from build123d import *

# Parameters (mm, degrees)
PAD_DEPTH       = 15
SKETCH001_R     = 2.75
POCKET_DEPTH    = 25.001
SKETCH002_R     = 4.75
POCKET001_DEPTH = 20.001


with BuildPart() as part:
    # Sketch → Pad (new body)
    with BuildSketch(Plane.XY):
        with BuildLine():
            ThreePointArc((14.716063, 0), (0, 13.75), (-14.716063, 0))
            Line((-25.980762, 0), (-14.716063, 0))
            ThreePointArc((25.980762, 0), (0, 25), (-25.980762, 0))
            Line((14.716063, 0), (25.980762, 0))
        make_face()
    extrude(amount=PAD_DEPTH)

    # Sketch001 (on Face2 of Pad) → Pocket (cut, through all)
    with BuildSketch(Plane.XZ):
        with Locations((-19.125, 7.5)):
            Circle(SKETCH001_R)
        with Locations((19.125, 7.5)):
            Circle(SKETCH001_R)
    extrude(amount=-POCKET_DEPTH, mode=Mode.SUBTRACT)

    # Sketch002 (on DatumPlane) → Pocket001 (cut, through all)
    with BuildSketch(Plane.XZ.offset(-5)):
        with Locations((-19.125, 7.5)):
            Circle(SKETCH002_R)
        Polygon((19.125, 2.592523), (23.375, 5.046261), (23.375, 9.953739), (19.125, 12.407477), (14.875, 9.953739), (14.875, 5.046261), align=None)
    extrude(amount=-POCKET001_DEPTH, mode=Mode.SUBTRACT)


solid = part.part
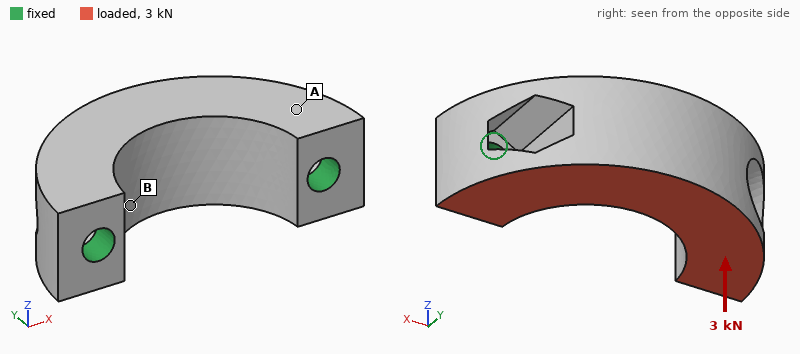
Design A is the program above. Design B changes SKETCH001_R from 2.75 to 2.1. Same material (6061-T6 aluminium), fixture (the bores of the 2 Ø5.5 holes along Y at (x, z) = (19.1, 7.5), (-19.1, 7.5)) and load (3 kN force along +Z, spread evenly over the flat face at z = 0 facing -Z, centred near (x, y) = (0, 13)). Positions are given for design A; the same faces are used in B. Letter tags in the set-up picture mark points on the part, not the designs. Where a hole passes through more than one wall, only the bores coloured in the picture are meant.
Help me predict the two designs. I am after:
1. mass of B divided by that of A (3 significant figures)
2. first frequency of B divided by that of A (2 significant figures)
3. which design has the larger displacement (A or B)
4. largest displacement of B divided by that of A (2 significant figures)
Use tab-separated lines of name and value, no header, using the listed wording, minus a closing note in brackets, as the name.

mass of B divided by that of A	1.01
first frequency of B divided by that of A	0.86
which design has the larger displacement	B
largest displacement of B divided by that of A	1.3
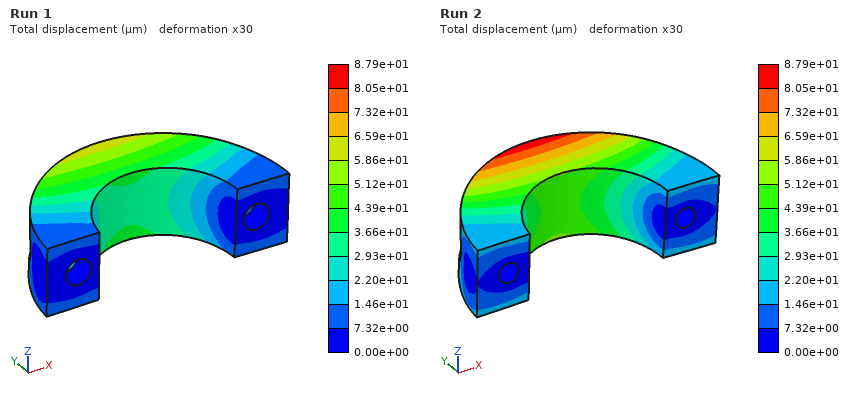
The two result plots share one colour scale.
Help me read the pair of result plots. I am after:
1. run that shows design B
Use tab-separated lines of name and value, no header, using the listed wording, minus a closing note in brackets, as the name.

run that shows design B	Run 2
